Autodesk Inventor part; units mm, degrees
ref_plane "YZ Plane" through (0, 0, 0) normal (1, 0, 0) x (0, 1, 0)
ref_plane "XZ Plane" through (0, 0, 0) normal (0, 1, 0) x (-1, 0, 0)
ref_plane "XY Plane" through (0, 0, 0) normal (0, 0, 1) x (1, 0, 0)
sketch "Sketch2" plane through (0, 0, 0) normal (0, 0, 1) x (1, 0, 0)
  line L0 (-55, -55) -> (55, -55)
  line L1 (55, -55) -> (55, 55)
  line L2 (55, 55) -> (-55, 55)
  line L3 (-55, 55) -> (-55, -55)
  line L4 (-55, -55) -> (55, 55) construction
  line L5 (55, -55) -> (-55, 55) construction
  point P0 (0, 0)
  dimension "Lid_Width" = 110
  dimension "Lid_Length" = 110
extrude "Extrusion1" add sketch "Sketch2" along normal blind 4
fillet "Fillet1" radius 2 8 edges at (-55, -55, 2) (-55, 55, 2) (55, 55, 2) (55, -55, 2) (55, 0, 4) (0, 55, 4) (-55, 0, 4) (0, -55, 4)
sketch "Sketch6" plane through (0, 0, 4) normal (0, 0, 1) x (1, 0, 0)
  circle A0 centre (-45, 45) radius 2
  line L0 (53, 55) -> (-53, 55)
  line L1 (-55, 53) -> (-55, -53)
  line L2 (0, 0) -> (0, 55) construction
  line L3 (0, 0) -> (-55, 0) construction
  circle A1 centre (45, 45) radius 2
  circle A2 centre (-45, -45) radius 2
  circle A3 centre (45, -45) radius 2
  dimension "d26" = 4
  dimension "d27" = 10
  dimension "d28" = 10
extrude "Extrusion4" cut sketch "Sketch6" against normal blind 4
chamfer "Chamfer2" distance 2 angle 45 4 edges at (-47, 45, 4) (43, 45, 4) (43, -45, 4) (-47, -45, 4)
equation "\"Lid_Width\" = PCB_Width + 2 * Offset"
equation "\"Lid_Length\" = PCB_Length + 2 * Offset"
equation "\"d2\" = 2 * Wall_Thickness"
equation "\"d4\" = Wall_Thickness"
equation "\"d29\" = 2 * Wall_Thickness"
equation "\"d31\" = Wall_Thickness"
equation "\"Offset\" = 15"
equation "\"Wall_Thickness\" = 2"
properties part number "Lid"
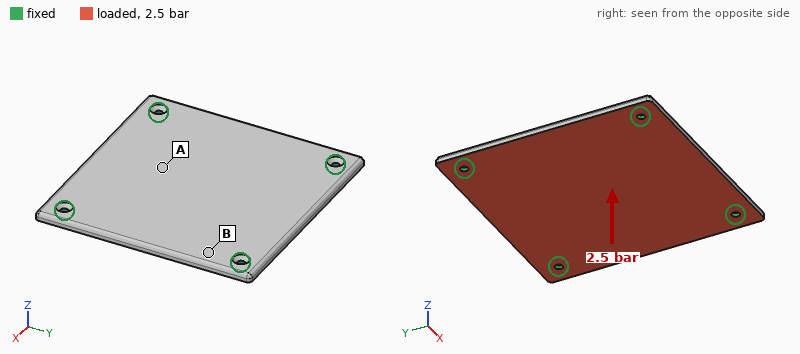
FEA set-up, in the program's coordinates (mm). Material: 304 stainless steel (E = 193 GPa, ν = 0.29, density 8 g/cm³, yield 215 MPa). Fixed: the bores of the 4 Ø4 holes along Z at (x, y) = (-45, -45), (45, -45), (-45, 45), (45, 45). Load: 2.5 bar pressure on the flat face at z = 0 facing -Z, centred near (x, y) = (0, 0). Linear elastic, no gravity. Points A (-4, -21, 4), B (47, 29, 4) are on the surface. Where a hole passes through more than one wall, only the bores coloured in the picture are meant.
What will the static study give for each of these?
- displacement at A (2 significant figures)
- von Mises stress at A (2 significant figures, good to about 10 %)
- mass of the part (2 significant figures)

0.13 mm
46 MPa
380 g
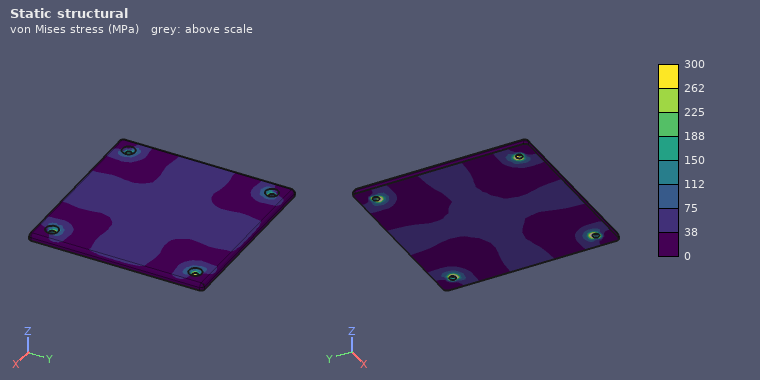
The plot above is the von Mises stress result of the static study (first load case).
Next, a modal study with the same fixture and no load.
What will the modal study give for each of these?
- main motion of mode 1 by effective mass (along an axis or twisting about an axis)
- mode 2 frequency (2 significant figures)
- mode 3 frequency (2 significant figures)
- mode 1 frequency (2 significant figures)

along Z
2400 Hz
2400 Hz
1400 Hz
